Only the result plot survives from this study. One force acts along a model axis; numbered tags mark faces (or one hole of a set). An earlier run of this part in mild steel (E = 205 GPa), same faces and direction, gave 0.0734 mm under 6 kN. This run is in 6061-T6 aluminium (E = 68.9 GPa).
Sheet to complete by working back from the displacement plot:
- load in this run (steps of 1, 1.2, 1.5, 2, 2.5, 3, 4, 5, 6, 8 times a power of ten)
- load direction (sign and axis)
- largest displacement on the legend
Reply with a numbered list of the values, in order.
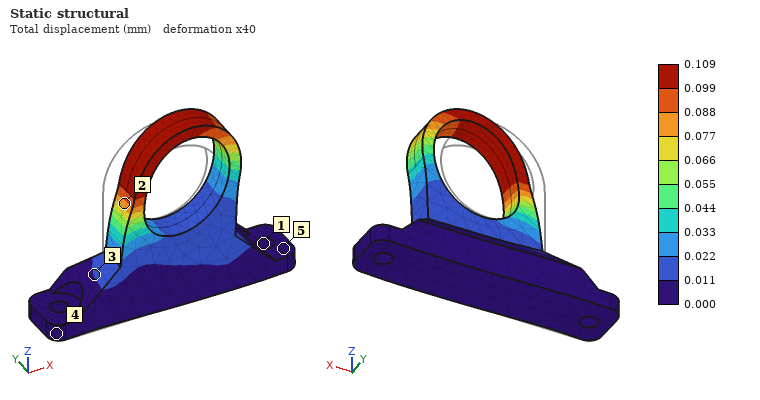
1. 3 kN
2. +X
3. 0.109 mm
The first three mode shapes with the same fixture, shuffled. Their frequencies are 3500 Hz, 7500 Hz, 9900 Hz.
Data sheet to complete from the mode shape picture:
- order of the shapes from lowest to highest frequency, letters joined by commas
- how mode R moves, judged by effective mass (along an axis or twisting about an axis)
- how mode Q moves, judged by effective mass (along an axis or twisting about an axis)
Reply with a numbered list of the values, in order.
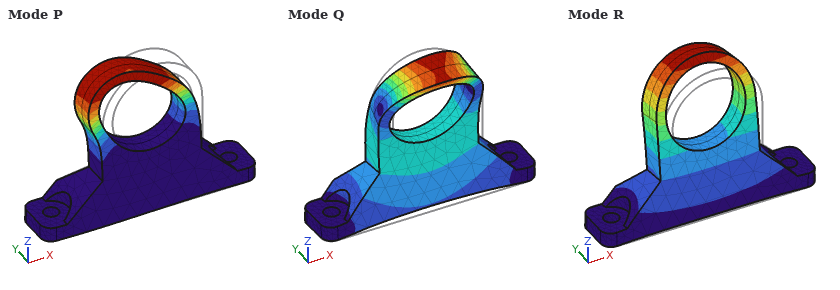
1. R, P, Q
2. along Y
3. along Y
